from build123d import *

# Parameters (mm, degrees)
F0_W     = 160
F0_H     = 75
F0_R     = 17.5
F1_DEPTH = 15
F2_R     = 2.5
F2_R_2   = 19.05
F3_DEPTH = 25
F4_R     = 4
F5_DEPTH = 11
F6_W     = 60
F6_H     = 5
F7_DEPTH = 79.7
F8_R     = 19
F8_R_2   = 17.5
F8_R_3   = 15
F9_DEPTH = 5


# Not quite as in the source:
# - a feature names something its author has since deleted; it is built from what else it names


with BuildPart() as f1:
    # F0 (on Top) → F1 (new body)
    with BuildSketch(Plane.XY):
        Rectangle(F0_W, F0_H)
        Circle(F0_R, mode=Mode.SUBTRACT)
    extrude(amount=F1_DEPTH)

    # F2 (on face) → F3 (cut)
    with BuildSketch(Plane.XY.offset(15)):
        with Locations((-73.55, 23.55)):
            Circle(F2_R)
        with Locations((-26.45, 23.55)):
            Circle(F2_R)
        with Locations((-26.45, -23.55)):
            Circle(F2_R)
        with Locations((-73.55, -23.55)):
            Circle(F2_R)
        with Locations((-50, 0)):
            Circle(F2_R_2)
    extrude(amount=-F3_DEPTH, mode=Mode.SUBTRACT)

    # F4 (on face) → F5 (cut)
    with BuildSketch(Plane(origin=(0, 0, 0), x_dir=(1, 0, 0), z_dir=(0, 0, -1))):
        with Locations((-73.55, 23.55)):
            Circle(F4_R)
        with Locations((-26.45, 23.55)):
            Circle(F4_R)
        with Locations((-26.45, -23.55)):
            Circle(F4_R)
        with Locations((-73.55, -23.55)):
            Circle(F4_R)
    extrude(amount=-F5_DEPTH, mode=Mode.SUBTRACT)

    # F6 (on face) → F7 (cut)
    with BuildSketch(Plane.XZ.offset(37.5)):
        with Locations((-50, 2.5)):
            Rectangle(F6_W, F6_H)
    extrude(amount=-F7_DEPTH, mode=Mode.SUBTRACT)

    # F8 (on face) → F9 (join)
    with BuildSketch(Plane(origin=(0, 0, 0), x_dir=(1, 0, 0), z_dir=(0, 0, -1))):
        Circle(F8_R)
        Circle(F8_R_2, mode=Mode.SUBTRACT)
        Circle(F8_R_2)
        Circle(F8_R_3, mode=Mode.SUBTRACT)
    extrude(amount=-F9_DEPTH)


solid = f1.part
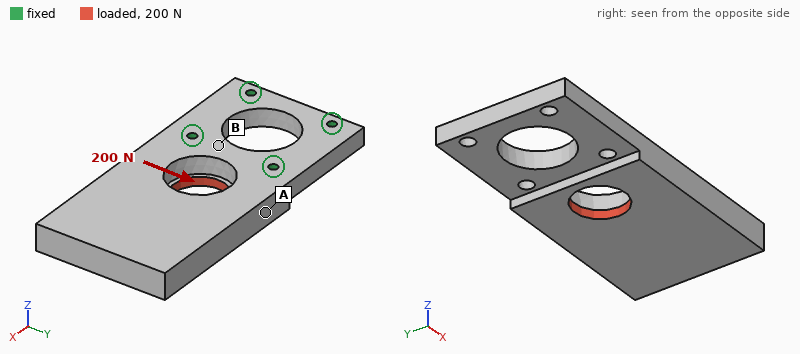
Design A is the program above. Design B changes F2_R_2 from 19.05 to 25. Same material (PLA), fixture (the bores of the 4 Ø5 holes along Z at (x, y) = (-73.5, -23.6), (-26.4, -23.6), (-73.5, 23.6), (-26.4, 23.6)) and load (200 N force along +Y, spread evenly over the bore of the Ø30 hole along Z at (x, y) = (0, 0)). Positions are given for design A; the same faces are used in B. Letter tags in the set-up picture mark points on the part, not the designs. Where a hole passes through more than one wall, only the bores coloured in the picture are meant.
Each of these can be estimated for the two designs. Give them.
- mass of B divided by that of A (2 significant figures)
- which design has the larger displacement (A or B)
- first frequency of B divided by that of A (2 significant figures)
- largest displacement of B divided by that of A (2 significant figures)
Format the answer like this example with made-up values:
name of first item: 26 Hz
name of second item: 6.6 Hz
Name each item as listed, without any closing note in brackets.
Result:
mass of B divided by that of A: 0.94
which design has the larger displacement: B
first frequency of B divided by that of A: 0.92
largest displacement of B divided by that of A: 1.1
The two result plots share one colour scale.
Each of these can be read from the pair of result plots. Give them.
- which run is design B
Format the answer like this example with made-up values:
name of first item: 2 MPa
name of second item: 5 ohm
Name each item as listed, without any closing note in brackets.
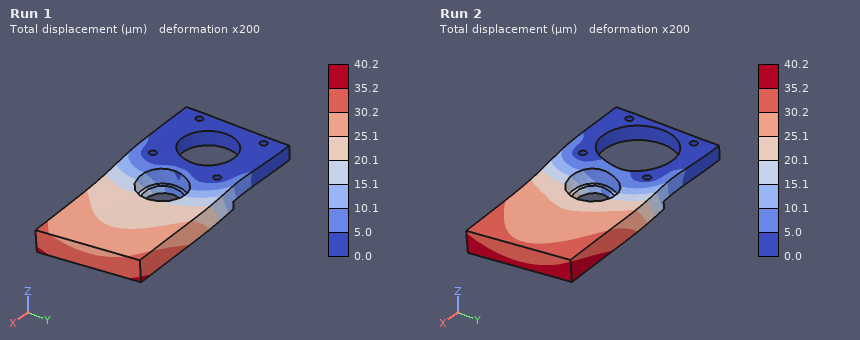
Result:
which run is design B: Run 2
